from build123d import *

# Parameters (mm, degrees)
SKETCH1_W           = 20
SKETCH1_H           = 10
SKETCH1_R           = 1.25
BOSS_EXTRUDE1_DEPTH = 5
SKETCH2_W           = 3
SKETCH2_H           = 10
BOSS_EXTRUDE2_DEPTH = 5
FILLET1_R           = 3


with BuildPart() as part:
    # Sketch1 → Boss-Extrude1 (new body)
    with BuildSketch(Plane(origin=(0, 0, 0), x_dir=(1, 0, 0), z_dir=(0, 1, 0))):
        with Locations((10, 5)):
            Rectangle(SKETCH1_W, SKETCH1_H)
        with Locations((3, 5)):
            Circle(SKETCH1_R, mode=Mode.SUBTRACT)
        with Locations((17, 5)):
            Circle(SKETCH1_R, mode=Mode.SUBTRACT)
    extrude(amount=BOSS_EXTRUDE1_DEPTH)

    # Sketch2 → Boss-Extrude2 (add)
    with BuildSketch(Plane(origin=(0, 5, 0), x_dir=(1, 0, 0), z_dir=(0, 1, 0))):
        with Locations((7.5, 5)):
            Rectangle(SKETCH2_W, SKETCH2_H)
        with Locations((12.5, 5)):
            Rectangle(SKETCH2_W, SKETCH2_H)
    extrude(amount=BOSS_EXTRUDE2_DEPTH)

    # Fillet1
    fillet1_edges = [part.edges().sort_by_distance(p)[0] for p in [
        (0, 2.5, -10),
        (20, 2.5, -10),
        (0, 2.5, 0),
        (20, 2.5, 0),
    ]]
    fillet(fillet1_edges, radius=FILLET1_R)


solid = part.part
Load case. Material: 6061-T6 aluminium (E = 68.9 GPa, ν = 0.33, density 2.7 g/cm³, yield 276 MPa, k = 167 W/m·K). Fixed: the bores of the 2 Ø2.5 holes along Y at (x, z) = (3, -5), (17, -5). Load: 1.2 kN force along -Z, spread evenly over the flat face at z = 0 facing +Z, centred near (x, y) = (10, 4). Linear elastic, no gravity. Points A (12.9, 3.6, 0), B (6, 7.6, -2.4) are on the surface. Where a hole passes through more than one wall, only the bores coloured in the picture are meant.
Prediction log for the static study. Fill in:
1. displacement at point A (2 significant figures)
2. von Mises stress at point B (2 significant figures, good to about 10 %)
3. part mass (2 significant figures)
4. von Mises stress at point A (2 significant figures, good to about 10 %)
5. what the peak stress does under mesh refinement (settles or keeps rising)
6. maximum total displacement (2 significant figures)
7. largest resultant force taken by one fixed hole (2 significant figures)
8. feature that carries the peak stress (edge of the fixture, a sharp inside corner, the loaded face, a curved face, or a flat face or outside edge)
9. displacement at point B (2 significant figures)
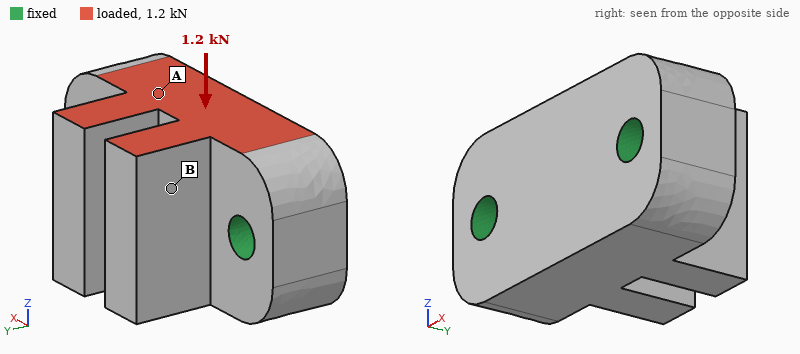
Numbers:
4.0 µm
12 MPa
3.3 g
29 MPa
keeps rising
8.6 µm
610 N
edge of the fixture
5.8 µm
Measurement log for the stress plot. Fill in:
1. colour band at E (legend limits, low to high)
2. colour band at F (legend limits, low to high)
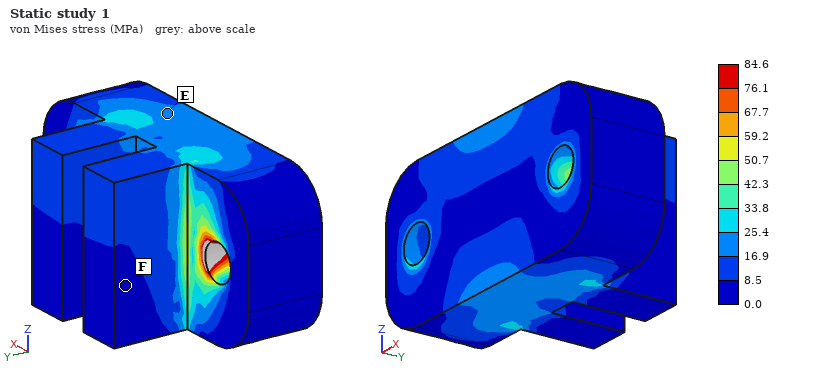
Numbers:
16.9 to 25.4 MPa
0.0 to 8.5 MPa
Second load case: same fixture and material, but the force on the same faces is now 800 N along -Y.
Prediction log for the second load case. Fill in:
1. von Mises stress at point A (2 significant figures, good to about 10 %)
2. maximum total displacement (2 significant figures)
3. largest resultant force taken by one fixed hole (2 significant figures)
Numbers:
21 MPa
12 µm
400 N
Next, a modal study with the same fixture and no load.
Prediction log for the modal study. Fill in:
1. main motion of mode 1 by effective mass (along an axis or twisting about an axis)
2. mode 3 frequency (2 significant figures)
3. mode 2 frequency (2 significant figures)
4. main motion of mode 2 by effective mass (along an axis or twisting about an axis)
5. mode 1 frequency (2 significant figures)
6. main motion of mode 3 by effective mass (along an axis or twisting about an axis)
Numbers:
along Z
58 kHz
50 kHz
along Y
42 kHz
along X
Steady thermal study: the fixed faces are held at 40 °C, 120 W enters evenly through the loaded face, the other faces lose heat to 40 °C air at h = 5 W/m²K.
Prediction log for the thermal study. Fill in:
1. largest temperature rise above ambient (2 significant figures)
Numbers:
63 K
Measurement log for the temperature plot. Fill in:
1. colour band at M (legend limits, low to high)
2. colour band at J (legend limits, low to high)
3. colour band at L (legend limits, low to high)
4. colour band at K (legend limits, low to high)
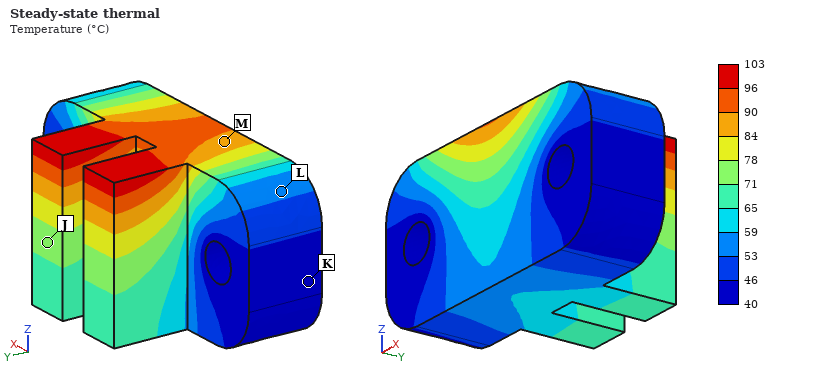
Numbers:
84 to 90 °C
71 to 78 °C
53 to 59 °C
40 to 46 °C
